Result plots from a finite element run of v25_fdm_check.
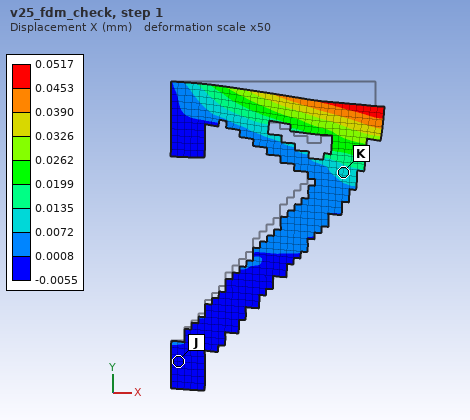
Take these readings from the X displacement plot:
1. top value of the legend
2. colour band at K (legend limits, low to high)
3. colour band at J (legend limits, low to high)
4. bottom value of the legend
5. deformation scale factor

0.0517 mm
0.0072 to 0.0135 mm
-0.0055 to 0.0008 mm
-0.0055 mm
50
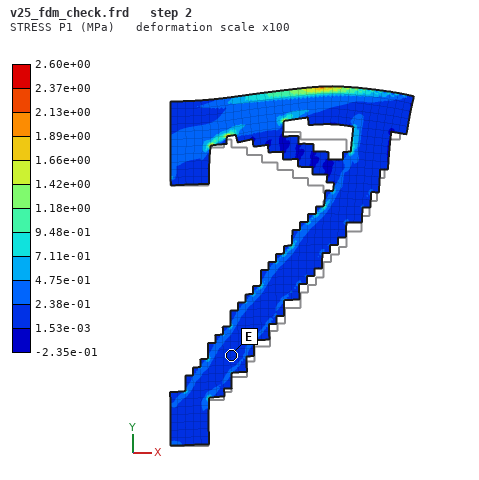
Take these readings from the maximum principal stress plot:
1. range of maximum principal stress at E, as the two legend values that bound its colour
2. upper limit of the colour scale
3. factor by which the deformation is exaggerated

1.53e-03 to 2.38e-01 MPa
2.60e+00 MPa
100
